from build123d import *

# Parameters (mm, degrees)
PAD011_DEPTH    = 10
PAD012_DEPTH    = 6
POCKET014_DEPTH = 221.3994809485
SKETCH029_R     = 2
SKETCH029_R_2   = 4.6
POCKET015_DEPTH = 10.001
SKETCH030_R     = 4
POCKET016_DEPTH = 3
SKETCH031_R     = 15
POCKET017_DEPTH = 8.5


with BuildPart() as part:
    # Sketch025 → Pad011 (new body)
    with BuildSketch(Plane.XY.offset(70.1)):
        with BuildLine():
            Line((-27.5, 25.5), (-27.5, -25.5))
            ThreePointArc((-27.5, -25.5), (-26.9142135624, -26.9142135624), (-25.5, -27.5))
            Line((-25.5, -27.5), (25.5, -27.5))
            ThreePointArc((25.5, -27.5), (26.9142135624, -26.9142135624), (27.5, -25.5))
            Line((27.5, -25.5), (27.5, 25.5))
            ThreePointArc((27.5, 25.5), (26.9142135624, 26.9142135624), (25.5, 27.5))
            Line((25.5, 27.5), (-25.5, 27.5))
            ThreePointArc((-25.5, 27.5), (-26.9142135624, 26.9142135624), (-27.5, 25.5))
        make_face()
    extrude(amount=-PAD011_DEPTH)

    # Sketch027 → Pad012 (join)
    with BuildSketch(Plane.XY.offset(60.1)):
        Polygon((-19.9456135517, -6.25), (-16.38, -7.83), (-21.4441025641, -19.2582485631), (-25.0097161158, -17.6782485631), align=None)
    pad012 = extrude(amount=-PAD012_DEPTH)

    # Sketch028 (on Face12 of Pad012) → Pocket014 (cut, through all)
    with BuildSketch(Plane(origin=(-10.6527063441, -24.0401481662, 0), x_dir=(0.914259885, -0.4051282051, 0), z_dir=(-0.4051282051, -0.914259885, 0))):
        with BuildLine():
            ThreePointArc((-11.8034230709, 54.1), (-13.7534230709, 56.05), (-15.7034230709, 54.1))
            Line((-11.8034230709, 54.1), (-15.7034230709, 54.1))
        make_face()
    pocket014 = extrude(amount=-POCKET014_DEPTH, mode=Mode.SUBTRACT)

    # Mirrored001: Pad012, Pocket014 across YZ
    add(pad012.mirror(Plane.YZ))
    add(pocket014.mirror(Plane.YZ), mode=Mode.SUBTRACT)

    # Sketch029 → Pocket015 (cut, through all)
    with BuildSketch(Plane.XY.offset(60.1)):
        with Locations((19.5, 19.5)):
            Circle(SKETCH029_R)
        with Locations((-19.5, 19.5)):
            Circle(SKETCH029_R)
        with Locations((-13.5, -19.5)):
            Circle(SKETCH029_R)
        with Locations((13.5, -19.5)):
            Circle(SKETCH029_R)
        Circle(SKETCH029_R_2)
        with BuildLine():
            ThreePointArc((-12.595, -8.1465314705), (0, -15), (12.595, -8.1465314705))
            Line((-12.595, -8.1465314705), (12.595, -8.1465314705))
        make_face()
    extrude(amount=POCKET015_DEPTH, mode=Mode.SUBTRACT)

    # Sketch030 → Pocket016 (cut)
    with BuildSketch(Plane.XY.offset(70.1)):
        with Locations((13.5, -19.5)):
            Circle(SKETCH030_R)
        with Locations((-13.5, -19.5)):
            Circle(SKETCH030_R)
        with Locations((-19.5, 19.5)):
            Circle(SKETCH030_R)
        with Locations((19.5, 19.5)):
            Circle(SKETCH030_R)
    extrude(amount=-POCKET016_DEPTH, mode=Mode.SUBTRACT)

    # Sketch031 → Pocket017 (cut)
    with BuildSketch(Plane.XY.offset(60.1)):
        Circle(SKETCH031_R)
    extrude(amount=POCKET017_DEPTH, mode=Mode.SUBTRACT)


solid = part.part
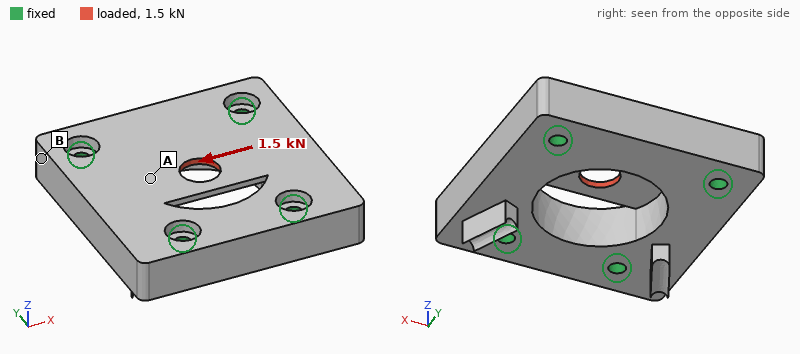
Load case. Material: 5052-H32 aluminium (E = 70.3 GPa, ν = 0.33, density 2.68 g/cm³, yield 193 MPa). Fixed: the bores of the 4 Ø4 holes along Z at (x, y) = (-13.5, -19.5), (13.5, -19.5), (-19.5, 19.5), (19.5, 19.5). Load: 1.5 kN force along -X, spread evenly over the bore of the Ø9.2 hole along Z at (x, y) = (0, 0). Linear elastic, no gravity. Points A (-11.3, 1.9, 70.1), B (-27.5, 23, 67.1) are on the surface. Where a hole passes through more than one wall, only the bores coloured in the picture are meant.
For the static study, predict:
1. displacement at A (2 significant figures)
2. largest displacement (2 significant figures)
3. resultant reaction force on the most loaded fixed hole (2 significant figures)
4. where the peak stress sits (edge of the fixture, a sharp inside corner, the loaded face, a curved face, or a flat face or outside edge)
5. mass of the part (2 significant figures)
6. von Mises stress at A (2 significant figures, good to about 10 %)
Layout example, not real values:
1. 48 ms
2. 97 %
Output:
1. 5.3 µm
2. 10 µm
3. 470 N
4. the loaded face
5. 63 g
6. 19 MPa
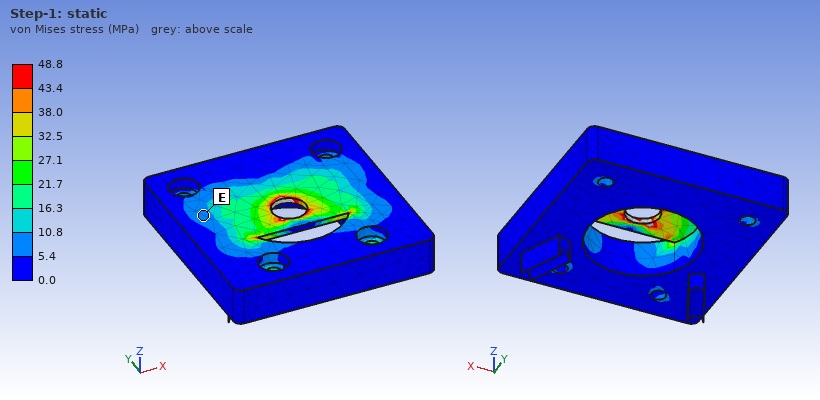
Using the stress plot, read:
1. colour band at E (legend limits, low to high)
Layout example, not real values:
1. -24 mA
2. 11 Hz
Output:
1. 5.4 to 10.8 MPa
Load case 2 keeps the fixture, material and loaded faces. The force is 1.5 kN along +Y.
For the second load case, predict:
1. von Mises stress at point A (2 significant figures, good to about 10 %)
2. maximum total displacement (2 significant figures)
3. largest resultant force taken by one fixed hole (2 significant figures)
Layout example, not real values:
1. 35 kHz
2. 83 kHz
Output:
1. 28 MPa
2. 20 µm
3. 580 N
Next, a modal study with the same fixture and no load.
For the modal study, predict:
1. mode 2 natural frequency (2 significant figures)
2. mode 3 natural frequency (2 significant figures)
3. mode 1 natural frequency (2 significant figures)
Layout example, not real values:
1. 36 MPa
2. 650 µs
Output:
1. 18 kHz
2. 19 kHz
3. 12 kHz
